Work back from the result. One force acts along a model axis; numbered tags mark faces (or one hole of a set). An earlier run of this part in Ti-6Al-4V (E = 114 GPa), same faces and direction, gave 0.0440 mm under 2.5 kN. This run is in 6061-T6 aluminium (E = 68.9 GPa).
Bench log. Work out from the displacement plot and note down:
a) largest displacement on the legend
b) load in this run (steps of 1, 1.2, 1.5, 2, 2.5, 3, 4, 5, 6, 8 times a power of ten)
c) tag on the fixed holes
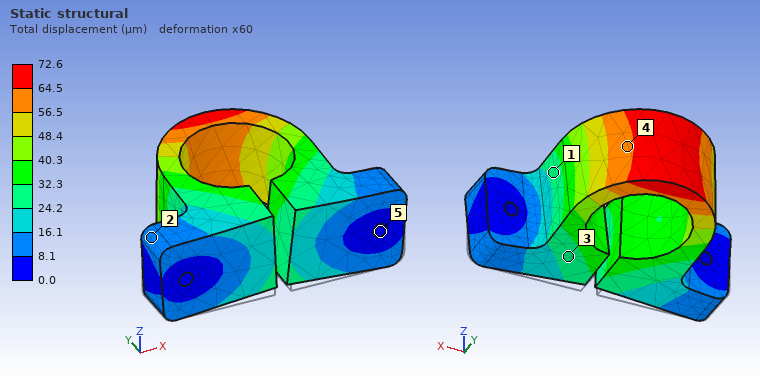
72.6 µm
2.5 kN
5
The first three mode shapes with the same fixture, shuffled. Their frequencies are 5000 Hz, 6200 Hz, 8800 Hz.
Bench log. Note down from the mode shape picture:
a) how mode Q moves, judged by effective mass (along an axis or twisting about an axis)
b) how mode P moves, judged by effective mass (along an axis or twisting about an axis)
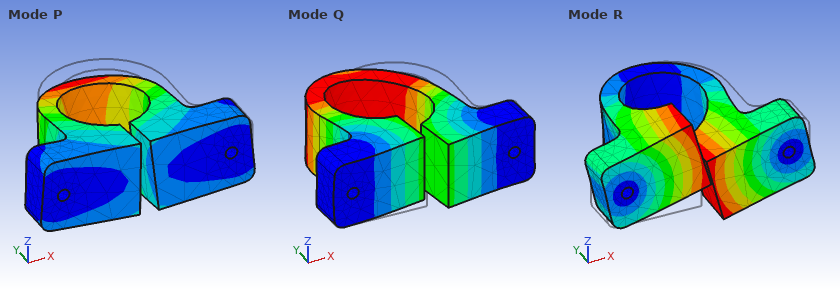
along X
along Z
